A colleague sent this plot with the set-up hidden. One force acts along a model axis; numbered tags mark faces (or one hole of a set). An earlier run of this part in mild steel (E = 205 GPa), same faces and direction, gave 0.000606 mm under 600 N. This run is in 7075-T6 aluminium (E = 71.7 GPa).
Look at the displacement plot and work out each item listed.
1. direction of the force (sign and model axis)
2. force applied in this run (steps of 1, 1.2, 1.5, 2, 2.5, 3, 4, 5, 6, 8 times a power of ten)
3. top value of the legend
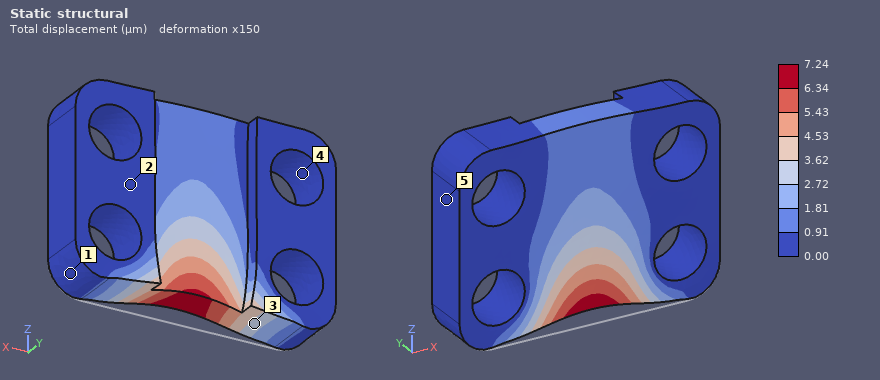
+Z
2.5 kN
7.24 µm
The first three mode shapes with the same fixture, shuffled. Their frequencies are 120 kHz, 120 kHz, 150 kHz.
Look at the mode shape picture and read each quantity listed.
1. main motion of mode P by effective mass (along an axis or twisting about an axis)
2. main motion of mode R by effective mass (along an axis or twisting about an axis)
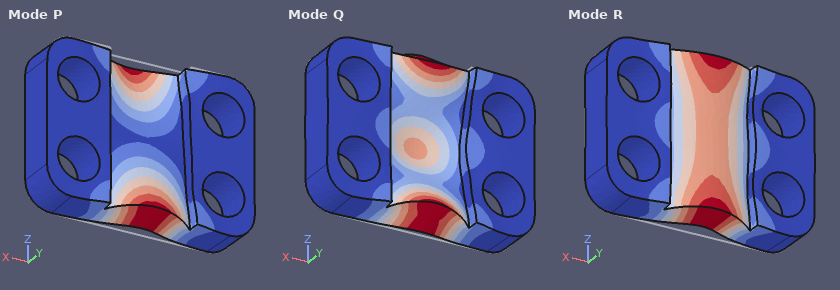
twisting about X
along Y
